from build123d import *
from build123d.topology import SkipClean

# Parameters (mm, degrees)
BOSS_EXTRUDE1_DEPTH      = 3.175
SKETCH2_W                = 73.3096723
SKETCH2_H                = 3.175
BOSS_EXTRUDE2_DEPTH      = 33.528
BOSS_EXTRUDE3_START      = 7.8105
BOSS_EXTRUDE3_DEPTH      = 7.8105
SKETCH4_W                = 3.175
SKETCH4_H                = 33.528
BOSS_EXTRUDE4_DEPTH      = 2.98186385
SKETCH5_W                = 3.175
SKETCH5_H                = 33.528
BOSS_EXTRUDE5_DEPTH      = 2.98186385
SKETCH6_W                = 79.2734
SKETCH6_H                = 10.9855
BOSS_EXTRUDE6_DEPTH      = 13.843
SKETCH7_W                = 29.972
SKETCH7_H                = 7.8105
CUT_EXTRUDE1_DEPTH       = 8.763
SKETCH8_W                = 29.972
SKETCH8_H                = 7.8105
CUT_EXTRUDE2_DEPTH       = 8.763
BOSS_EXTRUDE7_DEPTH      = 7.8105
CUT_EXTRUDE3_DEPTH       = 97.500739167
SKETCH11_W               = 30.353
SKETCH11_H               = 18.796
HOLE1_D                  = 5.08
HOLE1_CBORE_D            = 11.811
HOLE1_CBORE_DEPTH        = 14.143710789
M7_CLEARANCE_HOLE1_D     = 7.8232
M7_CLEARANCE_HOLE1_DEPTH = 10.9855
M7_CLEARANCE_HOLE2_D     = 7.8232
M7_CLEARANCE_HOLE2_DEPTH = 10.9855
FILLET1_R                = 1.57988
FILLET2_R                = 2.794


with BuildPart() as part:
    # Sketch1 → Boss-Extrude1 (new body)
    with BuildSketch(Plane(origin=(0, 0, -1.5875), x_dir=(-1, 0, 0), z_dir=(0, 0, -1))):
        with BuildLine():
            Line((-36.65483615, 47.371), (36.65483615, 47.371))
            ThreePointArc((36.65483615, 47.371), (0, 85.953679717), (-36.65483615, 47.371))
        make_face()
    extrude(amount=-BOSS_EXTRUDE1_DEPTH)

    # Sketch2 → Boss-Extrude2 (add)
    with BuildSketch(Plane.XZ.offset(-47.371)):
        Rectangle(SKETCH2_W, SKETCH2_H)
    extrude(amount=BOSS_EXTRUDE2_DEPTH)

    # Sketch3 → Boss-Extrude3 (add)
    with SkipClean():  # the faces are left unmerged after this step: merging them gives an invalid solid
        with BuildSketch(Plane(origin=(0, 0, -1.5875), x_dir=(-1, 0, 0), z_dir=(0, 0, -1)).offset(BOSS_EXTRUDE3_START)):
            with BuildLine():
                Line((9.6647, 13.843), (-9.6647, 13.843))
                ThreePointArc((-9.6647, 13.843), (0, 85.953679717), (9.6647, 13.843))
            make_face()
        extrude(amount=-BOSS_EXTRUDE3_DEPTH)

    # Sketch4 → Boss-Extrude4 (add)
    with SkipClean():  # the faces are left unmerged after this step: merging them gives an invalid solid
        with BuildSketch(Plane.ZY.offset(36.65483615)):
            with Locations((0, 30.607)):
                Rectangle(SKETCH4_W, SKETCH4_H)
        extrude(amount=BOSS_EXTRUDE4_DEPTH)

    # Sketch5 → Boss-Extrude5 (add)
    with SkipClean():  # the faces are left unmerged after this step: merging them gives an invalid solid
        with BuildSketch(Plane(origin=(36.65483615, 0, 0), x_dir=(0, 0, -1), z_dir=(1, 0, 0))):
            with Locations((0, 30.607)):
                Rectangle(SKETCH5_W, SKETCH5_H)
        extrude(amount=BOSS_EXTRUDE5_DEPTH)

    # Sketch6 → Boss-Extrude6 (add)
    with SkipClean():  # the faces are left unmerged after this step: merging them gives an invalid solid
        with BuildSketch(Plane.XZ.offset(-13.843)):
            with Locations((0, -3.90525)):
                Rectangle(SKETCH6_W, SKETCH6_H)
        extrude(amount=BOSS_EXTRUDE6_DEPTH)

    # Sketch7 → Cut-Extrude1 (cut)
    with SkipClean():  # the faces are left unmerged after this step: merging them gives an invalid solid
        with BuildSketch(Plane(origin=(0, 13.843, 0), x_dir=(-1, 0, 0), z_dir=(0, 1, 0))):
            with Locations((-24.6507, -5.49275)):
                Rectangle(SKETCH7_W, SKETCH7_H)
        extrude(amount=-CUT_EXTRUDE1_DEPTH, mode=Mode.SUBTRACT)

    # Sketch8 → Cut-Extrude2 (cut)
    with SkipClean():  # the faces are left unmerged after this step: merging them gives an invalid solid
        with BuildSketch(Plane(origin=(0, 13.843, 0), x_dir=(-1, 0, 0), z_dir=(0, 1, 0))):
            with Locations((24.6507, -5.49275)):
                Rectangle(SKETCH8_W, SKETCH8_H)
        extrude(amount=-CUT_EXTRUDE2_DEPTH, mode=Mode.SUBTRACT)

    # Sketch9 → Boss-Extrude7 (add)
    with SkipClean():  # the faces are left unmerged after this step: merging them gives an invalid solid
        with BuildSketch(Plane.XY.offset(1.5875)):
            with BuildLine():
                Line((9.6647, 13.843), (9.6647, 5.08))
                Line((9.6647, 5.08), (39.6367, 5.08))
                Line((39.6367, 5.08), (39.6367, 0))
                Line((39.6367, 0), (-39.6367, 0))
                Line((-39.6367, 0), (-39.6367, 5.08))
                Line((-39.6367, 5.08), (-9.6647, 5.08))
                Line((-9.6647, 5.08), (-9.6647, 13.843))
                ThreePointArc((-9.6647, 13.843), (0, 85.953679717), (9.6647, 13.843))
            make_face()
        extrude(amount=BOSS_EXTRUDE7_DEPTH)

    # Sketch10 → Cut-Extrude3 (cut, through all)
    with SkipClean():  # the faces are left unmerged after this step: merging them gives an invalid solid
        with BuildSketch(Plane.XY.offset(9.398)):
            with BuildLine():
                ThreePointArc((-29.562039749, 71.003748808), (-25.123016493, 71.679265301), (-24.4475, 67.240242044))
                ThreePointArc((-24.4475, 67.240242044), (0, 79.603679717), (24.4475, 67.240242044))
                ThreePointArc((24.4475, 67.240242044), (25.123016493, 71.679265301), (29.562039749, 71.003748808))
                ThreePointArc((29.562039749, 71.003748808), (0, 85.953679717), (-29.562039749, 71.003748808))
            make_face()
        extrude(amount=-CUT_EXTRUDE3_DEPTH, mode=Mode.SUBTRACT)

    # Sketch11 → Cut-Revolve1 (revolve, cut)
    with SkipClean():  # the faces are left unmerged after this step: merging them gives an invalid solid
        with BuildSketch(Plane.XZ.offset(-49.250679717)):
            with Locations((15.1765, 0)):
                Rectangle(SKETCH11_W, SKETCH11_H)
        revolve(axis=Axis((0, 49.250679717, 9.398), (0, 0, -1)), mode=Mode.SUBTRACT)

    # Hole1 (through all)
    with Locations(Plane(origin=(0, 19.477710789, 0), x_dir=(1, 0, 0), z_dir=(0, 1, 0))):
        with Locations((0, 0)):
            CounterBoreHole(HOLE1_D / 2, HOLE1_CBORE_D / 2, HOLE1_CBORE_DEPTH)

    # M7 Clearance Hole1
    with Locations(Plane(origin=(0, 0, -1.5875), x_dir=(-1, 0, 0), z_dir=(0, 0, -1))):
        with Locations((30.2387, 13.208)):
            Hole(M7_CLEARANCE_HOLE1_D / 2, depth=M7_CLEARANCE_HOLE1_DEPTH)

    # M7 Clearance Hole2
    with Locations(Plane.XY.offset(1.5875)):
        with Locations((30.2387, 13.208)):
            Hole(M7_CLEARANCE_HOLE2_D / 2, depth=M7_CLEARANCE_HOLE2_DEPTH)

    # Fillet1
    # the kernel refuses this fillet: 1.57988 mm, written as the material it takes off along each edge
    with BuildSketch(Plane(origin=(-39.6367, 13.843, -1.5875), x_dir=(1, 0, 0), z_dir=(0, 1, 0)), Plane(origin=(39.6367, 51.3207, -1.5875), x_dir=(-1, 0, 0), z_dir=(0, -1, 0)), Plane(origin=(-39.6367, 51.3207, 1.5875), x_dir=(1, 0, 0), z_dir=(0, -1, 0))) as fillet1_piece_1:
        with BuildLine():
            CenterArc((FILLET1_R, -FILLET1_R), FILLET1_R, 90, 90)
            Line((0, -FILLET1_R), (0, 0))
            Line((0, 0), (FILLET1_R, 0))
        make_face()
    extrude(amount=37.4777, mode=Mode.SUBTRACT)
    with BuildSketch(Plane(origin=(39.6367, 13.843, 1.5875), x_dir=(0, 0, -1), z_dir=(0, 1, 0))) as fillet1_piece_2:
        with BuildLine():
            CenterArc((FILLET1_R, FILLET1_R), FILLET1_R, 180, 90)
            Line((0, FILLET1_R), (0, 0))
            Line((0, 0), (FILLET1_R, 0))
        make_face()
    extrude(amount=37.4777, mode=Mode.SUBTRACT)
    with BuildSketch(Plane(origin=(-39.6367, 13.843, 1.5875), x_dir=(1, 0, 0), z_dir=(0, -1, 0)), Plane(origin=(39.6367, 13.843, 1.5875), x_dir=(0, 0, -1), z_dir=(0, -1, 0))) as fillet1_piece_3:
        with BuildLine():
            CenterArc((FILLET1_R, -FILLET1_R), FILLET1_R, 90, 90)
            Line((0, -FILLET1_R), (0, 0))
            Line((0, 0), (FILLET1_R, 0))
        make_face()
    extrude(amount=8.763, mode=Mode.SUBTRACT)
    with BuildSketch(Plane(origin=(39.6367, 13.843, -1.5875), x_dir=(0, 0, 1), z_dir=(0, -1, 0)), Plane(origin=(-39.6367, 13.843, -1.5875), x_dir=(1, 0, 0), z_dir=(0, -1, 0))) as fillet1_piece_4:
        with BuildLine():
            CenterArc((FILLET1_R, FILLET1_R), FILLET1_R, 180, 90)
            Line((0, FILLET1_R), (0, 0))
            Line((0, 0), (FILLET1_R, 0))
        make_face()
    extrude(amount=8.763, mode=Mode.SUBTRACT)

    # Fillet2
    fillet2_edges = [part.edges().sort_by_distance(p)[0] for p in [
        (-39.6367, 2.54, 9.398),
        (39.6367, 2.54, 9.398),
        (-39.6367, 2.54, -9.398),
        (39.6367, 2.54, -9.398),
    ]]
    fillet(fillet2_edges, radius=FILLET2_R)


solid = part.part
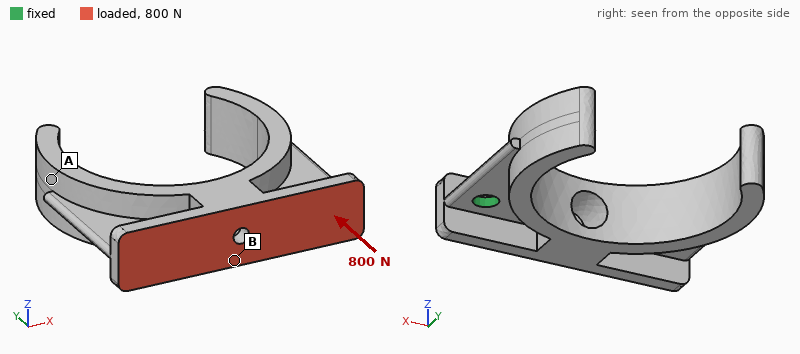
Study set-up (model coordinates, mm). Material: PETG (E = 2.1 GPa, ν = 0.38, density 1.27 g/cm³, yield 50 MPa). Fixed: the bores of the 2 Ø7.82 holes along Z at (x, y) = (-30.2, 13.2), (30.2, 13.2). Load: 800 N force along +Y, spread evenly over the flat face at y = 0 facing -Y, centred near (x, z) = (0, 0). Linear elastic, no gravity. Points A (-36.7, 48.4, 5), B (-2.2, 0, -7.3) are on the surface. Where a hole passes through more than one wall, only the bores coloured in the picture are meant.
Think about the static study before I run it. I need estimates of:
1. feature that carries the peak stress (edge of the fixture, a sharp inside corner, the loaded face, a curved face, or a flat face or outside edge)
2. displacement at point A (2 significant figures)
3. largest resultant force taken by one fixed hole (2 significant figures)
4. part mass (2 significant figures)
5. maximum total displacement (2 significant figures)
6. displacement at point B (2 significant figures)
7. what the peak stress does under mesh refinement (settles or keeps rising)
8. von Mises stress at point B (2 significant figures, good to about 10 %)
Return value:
edge of the fixture
0.14 mm
420 N
39 g
0.24 mm
0.11 mm
keeps rising
2.8 MPa
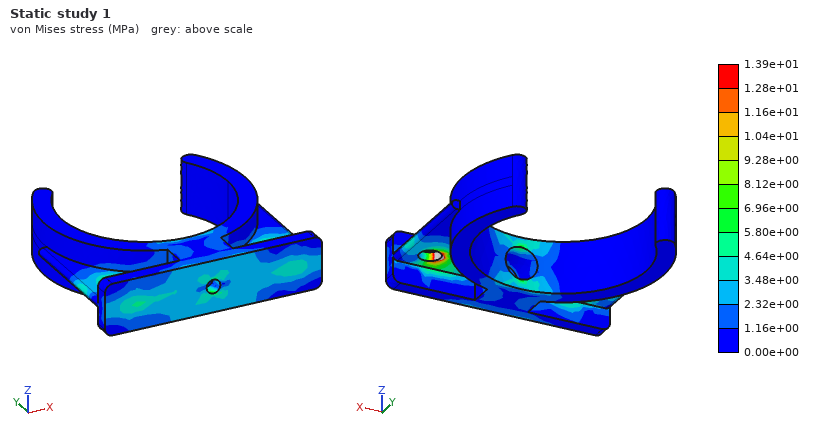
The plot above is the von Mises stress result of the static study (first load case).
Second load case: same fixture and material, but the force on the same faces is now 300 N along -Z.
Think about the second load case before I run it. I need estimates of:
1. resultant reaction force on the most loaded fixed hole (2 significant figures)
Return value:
150 N
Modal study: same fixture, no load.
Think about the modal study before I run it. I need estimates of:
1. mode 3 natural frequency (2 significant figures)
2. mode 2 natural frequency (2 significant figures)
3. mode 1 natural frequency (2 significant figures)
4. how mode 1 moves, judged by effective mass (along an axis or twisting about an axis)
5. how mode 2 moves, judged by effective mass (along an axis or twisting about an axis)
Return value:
720 Hz
490 Hz
340 Hz
along Z
twisting about Y
